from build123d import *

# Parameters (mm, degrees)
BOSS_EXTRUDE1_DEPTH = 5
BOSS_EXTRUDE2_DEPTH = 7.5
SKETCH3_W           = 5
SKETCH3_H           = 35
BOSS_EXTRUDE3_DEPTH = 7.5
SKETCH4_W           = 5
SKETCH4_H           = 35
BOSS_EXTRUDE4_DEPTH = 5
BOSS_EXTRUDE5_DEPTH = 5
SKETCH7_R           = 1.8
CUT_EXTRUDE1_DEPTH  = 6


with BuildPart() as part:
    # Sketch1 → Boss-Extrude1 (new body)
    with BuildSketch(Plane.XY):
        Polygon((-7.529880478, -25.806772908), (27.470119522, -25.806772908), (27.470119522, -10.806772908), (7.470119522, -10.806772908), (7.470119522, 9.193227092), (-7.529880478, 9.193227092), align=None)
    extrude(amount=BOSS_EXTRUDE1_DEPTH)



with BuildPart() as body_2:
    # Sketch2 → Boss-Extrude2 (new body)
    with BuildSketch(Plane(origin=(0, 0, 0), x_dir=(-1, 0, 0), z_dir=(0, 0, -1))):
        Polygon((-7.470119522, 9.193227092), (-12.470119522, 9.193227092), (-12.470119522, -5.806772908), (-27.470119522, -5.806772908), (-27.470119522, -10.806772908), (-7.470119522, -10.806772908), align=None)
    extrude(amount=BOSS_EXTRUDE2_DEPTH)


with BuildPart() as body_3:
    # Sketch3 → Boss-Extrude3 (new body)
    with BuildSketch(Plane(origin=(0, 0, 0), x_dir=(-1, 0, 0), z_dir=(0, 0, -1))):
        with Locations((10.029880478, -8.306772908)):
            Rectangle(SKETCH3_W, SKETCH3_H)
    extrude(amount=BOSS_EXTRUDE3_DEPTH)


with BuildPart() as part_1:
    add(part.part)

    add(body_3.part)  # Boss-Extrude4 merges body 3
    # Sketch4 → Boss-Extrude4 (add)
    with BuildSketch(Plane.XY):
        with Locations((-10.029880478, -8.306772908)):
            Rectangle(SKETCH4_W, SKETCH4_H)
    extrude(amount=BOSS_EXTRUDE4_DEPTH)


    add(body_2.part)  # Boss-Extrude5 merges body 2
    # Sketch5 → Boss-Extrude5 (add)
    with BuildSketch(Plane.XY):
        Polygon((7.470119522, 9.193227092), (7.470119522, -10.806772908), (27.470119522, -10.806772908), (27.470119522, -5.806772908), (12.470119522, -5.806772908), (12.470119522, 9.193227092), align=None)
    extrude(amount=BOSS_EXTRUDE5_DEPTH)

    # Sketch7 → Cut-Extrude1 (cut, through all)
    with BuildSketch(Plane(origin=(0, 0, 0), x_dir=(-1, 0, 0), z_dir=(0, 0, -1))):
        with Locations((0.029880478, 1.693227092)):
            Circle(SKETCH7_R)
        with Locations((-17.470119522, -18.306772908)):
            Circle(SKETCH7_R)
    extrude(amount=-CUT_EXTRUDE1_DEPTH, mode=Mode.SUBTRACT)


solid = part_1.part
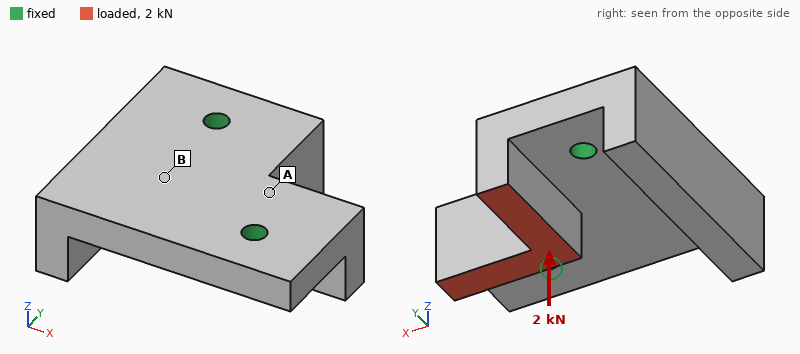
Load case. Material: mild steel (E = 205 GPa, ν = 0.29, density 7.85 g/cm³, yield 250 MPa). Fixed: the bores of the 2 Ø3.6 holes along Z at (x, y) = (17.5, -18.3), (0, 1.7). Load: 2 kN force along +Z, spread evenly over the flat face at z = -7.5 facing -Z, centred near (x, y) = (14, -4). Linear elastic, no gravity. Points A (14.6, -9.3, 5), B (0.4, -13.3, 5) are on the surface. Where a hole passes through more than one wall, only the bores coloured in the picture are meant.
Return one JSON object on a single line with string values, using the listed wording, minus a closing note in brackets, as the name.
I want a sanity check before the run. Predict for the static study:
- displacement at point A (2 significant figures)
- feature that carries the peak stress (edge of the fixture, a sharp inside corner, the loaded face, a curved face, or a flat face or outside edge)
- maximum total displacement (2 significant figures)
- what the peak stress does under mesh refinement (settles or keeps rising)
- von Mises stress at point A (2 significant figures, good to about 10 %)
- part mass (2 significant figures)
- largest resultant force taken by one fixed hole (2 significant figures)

{"displacement at point A": "5.7 µm", "feature that carries the peak stress": "edge of the fixture", "maximum total displacement": "19 µm", "what the peak stress does under mesh refinement": "keeps rising", "von Mises stress at point A": "35 MPa", "part mass": "66 g", "largest resultant force taken by one fixed hole": "1.1 kN"}
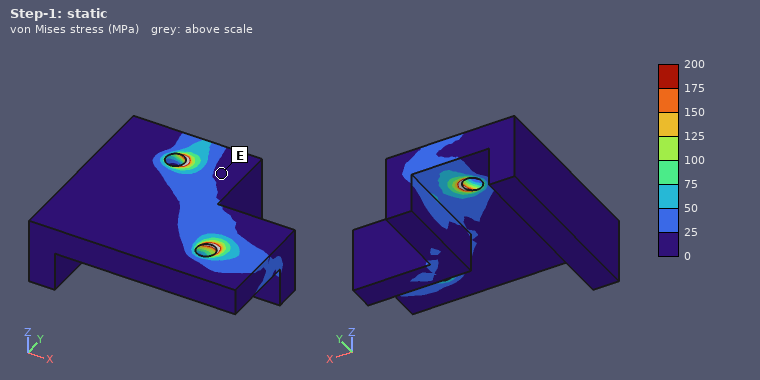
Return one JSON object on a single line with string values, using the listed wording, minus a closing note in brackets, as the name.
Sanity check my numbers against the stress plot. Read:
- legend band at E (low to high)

{"legend band at E": "0 to 25 MPa"}
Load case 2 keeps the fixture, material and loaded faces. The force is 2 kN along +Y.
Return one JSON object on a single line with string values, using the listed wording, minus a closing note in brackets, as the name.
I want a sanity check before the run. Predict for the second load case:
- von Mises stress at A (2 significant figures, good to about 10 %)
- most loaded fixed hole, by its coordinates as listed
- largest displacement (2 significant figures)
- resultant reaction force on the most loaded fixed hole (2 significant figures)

{"von Mises stress at A": "49 MPa", "most loaded fixed hole, by its coordinates as listed": "(17.5, -18.3)", "largest displacement": "25 µm", "resultant reaction force on the most loaded fixed hole": "1.3 kN"}
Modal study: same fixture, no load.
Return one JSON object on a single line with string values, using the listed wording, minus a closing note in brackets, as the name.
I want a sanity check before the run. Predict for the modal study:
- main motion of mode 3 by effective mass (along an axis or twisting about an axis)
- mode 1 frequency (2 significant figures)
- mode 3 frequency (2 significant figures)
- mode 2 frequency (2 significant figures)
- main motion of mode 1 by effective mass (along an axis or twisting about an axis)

{"main motion of mode 3 by effective mass": "along Z", "mode 1 frequency": "6400 Hz", "mode 3 frequency": "15 kHz", "mode 2 frequency": "14 kHz", "main motion of mode 1 by effective mass": "along Z"}
